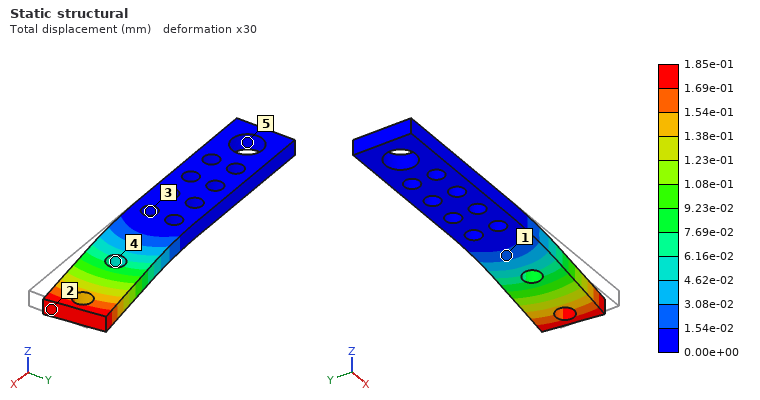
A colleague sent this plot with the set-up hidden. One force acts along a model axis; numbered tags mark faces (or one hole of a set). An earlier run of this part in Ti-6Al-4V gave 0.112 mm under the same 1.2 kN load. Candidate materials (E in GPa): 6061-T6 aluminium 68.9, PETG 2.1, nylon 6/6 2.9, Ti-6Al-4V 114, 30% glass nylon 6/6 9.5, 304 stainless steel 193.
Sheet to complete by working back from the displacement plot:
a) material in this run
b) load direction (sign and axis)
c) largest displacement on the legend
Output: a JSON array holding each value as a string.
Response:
["6061-T6 aluminium", "+Y", "1.85e-01 mm"]
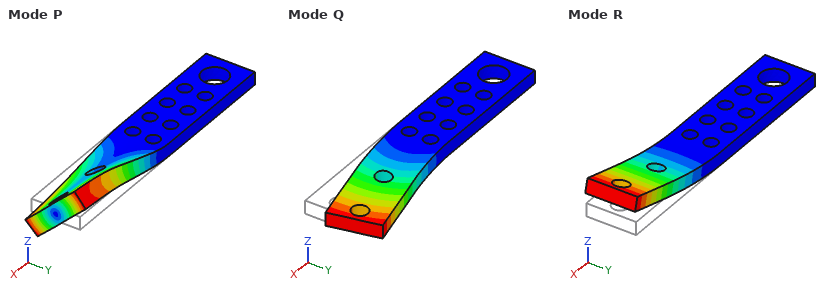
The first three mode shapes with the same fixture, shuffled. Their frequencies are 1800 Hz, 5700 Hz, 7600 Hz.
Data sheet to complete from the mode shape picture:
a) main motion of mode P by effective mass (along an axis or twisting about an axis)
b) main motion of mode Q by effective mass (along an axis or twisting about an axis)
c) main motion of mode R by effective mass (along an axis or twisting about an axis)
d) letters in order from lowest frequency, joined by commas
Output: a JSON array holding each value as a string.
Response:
["twisting about X", "along Y", "along Z", "R, Q, P"]
